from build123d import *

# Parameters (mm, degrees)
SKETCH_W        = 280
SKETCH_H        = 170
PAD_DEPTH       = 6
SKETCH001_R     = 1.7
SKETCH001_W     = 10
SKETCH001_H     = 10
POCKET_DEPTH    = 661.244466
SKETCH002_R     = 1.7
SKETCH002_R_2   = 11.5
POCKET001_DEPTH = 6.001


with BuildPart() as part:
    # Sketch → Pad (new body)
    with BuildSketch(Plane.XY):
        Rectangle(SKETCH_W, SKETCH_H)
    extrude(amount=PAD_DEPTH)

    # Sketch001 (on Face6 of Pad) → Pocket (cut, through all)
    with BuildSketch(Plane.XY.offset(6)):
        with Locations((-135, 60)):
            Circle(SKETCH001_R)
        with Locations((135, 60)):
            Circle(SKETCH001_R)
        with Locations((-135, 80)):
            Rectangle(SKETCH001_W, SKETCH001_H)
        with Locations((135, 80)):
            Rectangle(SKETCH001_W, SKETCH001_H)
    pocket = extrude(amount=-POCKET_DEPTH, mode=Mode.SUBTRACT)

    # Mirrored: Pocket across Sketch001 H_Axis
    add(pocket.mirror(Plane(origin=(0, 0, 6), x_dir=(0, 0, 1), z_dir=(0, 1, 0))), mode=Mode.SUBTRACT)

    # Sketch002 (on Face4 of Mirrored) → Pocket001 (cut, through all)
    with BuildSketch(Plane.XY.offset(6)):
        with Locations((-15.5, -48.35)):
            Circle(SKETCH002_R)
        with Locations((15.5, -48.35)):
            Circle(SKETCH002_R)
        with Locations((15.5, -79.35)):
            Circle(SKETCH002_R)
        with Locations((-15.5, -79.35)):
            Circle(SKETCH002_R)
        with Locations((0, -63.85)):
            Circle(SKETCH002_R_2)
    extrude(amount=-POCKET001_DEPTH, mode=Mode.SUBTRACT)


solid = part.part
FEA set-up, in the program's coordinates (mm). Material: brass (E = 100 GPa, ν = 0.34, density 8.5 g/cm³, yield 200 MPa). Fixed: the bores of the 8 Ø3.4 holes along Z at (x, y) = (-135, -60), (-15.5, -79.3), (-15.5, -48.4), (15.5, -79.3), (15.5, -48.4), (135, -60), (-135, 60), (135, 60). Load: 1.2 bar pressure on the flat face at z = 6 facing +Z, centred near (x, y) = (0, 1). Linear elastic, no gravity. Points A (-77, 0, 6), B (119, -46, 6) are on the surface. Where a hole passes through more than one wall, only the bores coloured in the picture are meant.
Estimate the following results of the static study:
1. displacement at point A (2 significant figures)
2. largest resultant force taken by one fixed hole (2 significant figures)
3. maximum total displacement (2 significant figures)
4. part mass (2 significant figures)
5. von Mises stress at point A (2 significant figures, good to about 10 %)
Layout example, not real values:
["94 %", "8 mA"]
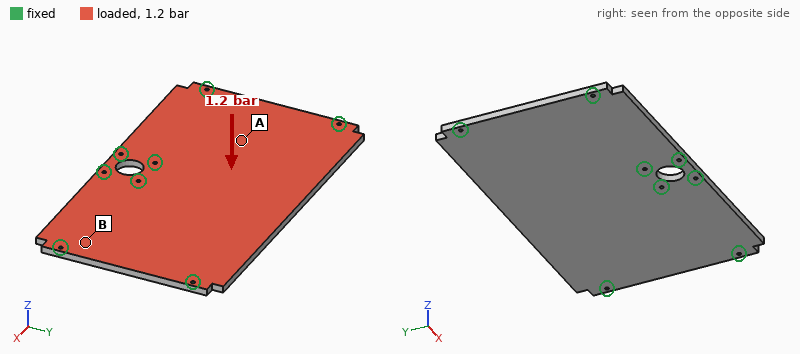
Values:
["0.21 mm", "1.5 kN", "0.87 mm", "2.4 kg", "31 MPa"]
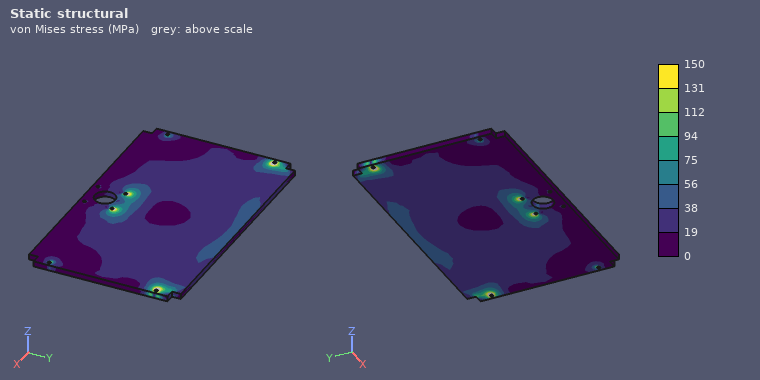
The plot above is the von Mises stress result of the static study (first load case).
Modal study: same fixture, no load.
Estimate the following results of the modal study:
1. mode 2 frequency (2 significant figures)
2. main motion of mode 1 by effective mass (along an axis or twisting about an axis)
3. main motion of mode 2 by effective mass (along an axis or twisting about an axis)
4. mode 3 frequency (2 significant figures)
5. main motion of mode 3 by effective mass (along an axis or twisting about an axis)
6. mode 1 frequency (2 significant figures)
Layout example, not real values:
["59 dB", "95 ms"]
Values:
["750 Hz", "along Z", "twisting about Y", "960 Hz", "along Z", "360 Hz"]
